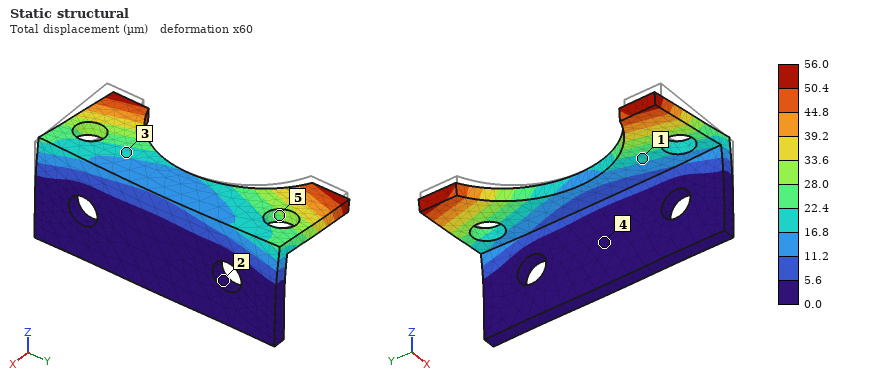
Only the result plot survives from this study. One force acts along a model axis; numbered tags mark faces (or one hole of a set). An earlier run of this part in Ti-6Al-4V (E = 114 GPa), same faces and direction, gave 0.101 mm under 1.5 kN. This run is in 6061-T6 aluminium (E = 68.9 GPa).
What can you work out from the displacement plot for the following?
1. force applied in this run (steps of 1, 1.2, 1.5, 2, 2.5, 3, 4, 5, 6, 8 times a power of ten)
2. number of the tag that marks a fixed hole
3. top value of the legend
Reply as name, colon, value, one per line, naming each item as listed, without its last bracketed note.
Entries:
force applied in this run: 500 N
number of the tag that marks a fixed hole: 2
top value of the legend: 56.0 µm
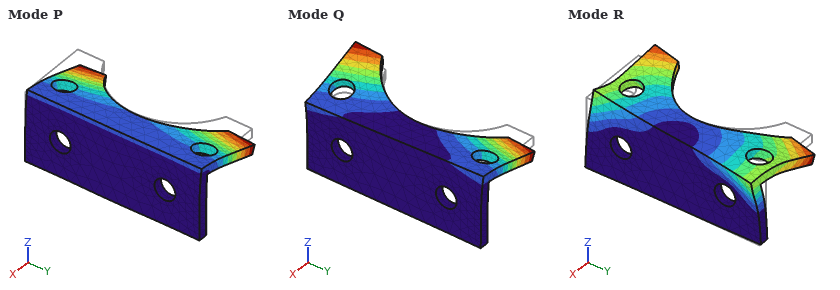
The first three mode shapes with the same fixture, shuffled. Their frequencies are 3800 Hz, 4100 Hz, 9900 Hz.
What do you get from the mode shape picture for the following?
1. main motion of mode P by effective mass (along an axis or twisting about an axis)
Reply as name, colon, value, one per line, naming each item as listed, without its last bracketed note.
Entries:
main motion of mode P by effective mass: along Z
